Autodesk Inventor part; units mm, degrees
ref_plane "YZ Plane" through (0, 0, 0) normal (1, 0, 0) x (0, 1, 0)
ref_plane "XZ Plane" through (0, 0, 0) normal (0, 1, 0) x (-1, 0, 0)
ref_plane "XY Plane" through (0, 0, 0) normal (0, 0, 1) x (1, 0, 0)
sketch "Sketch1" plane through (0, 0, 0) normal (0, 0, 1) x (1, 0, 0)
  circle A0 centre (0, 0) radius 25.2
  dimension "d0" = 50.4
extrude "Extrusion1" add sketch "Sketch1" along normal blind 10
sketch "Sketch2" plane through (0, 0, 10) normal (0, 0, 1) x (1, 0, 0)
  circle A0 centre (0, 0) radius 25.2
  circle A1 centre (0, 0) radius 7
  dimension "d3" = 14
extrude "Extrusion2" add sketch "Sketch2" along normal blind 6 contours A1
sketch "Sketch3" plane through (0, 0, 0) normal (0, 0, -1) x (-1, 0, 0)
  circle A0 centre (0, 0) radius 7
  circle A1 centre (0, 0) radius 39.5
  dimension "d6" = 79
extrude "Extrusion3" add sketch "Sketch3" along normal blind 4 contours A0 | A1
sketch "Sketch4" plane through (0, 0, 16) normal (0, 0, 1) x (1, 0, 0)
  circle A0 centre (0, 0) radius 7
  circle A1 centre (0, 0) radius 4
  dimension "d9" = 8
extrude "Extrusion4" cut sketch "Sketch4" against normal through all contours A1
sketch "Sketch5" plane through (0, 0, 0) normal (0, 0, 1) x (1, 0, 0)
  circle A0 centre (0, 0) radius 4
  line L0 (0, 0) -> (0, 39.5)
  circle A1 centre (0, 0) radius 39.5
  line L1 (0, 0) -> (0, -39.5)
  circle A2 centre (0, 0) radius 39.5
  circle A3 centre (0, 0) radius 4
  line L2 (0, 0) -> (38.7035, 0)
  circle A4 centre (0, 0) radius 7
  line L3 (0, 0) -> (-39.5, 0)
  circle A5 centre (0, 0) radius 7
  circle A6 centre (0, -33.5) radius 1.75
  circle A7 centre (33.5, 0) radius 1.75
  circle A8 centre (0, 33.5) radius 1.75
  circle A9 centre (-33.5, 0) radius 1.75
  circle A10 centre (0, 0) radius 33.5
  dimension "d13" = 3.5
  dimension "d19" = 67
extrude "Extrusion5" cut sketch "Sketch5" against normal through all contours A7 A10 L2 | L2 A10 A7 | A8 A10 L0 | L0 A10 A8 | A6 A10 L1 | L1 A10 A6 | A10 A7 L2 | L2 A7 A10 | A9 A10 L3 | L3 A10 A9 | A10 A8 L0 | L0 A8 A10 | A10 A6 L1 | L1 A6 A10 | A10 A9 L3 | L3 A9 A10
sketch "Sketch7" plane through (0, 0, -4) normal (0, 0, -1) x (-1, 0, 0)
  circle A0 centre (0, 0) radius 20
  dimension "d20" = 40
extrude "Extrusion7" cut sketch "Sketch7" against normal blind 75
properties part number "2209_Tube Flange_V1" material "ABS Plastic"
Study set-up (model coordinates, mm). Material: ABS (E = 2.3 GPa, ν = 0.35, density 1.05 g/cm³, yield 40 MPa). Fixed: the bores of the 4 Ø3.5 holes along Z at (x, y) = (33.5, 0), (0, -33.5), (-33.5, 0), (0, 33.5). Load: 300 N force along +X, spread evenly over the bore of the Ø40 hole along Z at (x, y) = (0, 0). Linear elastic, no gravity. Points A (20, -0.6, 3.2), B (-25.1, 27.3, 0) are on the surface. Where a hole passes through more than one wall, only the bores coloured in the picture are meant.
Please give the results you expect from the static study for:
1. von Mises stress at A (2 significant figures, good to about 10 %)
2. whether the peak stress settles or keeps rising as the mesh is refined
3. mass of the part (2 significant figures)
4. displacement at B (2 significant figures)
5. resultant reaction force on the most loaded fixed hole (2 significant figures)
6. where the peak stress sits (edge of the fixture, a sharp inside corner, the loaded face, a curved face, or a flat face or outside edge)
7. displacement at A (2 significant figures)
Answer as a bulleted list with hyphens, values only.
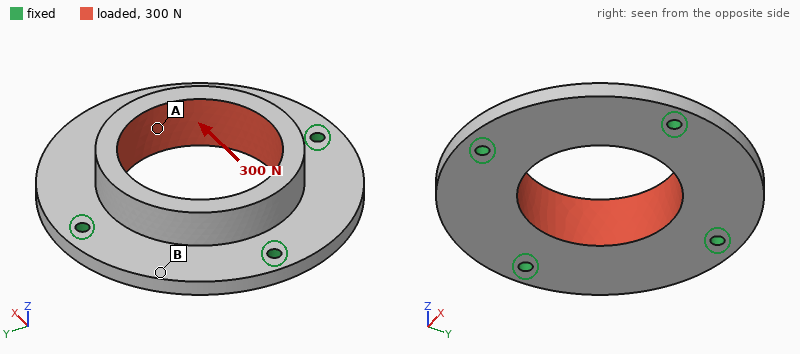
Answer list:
- 1.0 MPa
- keeps rising
- 23 g
- 18 µm
- 77 N
- edge of the fixture
- 11 µm
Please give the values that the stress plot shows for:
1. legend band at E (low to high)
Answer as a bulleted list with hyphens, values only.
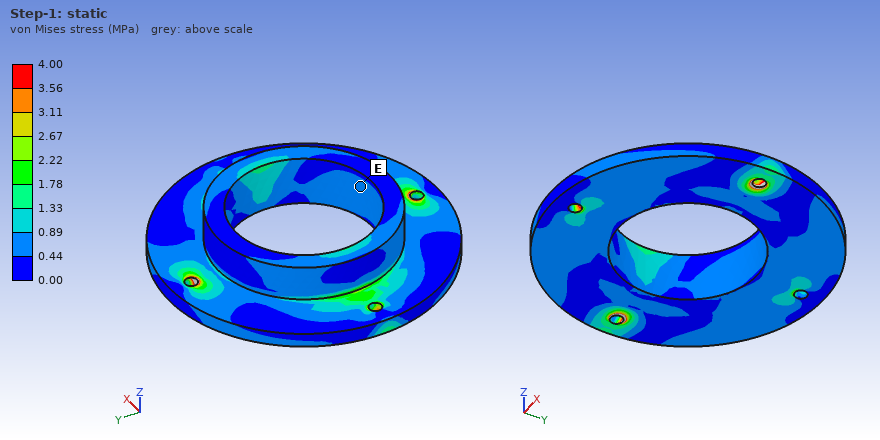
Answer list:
- 0.44 to 0.89 MPa
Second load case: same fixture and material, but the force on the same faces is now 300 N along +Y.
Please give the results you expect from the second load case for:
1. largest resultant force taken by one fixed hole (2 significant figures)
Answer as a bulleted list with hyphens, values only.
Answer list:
- 77 N
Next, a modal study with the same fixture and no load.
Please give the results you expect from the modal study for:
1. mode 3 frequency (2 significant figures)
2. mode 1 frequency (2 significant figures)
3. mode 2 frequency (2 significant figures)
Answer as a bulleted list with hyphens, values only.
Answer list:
- 2500 Hz
- 2300 Hz
- 2500 Hz
